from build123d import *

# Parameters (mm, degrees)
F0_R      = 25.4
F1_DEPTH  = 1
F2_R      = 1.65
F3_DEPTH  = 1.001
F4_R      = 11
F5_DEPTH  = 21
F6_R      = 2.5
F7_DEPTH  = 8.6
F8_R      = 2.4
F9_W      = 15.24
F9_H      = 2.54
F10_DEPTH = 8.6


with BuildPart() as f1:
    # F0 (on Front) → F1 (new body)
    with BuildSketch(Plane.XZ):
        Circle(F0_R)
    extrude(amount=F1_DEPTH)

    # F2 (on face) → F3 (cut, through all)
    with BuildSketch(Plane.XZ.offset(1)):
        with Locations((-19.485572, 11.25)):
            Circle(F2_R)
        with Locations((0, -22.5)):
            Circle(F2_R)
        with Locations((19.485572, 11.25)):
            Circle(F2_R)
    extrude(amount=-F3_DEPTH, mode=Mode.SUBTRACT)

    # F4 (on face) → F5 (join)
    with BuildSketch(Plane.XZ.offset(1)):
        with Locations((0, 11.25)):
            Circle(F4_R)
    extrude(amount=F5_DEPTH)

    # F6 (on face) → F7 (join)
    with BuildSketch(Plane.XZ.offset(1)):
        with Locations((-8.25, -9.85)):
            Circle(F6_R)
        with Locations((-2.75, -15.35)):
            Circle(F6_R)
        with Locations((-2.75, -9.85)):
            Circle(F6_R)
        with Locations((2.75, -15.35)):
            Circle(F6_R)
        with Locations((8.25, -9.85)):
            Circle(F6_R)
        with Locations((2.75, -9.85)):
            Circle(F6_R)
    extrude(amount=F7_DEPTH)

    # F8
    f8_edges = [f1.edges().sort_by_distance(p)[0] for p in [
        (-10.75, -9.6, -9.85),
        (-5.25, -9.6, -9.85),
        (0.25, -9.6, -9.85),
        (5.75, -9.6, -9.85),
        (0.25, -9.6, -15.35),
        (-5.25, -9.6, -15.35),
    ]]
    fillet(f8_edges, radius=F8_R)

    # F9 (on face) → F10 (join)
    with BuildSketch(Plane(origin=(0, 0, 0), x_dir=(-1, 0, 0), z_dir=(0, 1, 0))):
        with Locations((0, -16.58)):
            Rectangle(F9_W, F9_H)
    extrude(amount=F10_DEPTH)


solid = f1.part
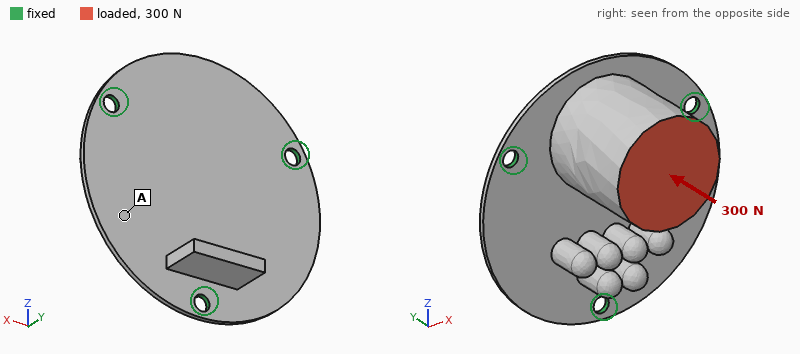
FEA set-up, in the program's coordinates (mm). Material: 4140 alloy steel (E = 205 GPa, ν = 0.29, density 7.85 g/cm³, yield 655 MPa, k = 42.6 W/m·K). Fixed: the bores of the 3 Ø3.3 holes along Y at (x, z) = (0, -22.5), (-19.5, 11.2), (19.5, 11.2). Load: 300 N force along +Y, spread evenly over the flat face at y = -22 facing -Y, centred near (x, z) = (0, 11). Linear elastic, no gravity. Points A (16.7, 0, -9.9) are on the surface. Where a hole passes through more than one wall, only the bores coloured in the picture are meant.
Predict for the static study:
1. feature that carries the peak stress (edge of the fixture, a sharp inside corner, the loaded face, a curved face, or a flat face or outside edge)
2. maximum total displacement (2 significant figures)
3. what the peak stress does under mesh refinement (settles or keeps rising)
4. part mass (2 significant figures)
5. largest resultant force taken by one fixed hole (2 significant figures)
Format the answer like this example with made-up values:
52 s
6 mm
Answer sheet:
edge of the fixture
48 µm
keeps rising
88 g
160 N
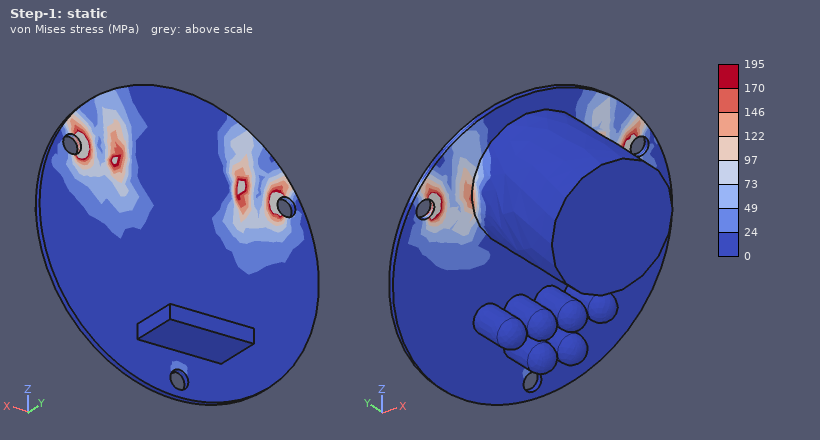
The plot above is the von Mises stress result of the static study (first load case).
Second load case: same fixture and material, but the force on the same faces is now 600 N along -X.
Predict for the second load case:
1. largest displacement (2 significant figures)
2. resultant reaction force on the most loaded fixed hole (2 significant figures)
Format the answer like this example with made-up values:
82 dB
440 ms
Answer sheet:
0.14 mm
490 N
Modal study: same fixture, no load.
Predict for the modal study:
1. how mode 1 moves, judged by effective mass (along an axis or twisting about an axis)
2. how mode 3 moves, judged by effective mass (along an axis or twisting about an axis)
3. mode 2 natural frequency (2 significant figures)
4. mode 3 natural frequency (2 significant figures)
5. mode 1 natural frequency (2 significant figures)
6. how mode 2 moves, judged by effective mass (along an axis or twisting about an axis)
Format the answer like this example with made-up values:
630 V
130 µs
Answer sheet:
along Z
along X
1900 Hz
2100 Hz
890 Hz
along Y
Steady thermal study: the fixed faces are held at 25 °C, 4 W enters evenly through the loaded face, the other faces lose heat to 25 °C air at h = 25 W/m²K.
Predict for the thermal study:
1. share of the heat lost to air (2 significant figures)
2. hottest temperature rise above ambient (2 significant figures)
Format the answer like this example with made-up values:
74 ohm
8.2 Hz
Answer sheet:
38 %
21 K
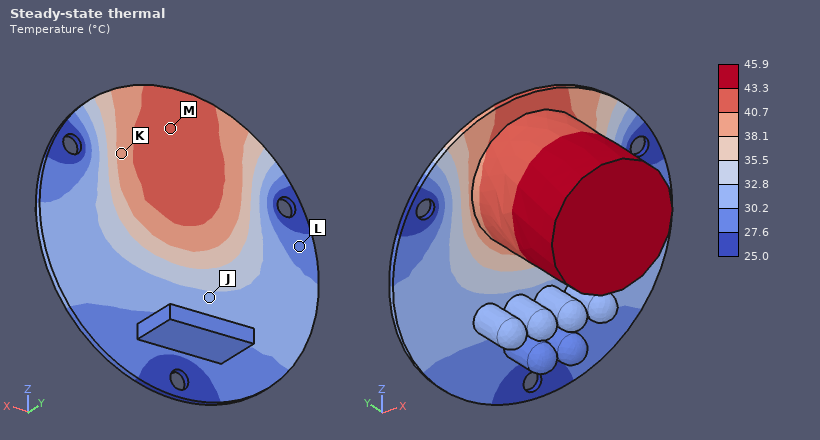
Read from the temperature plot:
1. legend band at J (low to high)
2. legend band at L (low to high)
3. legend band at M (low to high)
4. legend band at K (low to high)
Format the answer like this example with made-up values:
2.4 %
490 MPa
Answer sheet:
30.2 to 32.8 °C
27.6 to 30.2 °C
40.7 to 43.3 °C
38.1 to 40.7 °C
